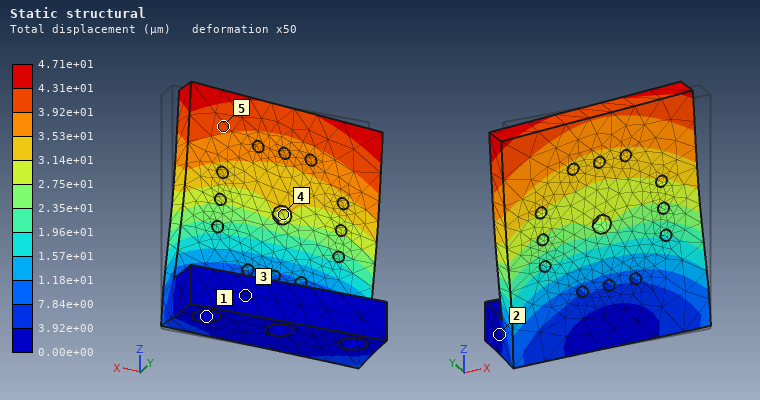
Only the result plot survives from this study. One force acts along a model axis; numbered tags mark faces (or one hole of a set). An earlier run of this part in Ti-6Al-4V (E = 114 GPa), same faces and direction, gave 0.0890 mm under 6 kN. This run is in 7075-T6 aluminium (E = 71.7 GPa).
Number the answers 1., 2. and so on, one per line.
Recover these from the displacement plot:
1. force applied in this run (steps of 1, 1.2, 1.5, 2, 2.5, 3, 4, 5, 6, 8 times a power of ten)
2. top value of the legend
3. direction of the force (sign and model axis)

1. 2 kN
2. 4.71e+01 µm
3. -X
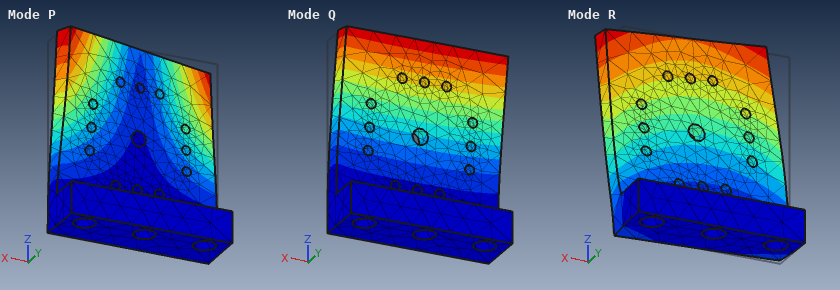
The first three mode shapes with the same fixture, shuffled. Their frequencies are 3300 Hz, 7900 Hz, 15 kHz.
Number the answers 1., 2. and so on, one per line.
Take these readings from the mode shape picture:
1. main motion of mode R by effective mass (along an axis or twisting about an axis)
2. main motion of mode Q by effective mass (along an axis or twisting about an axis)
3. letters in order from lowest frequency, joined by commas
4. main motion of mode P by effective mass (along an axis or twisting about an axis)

1. along X
2. along Y
3. Q, P, R
4. twisting about Z
